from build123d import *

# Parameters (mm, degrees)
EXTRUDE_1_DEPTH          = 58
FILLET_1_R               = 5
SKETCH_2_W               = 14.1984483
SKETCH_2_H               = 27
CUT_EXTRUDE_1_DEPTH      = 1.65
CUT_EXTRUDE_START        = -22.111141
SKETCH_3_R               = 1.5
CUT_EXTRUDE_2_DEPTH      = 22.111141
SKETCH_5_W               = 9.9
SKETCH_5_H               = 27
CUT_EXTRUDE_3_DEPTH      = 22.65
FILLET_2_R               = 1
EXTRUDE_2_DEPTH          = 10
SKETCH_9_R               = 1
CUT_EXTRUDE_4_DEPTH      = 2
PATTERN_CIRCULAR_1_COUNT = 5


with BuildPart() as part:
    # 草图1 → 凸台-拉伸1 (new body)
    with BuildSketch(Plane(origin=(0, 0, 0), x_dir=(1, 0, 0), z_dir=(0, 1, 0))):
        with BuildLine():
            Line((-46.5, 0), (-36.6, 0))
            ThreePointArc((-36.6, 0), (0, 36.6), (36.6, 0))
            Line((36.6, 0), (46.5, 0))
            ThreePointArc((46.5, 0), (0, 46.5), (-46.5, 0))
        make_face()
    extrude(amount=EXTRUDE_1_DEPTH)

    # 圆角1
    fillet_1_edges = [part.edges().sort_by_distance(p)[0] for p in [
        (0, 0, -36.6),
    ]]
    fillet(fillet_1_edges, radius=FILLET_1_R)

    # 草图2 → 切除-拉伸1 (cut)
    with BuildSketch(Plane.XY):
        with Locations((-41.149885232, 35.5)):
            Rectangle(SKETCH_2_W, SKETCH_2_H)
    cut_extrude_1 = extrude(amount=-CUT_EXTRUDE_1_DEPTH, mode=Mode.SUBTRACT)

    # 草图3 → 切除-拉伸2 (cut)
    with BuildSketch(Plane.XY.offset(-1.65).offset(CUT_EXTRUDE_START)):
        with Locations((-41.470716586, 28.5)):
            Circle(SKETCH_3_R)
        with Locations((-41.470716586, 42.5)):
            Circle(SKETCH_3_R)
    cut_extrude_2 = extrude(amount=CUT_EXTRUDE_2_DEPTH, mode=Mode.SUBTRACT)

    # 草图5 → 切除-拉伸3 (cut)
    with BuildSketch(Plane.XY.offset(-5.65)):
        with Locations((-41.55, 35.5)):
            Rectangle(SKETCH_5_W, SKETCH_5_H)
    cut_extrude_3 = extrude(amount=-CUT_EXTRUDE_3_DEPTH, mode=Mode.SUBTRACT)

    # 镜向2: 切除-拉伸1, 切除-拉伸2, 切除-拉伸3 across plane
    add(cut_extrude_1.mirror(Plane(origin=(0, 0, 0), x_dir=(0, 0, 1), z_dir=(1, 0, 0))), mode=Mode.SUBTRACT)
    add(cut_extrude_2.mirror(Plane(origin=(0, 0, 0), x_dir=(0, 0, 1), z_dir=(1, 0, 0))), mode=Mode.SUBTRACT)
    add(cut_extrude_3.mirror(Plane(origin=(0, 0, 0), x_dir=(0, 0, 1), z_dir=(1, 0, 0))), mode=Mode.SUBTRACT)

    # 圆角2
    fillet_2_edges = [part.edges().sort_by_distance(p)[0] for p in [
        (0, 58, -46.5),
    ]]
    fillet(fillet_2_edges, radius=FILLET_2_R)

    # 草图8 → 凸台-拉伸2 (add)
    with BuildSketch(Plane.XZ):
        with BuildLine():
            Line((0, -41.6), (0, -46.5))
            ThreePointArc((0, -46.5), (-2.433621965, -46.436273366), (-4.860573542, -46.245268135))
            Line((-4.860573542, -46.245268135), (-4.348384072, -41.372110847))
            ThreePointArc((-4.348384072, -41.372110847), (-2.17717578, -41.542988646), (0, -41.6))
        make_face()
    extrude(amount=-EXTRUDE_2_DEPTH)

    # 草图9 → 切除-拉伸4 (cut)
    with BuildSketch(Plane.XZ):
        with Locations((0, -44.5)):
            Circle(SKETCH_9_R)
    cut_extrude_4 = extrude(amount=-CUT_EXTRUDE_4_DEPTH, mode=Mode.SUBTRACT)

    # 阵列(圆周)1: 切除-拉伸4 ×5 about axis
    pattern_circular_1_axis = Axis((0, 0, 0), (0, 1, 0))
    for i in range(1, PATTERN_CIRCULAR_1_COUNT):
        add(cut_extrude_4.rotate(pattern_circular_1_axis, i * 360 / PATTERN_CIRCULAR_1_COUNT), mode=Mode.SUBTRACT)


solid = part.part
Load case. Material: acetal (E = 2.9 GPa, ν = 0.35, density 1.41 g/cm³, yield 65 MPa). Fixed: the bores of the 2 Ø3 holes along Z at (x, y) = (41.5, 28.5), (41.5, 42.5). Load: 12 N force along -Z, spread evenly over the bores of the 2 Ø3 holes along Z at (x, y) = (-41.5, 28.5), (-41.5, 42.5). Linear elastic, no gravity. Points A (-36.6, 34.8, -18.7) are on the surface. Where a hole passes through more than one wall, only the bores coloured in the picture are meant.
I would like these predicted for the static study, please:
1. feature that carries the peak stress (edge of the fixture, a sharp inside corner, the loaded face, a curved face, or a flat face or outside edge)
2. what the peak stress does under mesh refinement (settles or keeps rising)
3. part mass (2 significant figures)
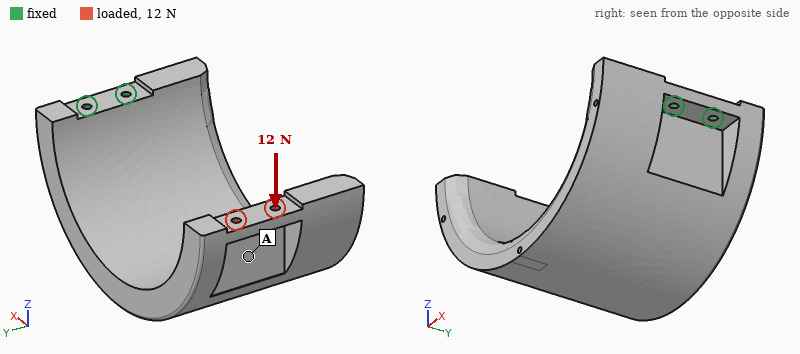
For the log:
edge of the fixture
keeps rising
93 g
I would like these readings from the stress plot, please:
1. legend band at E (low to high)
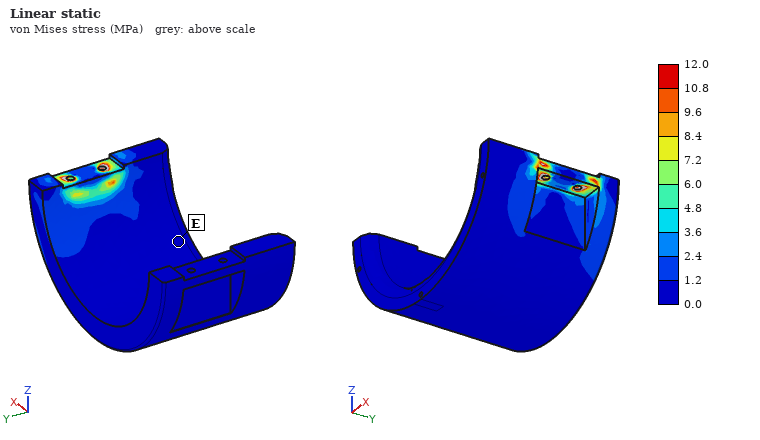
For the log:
0.0 to 1.2 MPa
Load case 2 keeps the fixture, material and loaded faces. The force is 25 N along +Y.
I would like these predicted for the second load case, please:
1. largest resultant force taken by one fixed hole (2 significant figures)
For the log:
100 N
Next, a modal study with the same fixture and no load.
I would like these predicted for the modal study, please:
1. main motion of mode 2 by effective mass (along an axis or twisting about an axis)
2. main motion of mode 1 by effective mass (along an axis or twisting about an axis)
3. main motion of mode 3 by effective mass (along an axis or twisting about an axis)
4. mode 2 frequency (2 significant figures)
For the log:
along Y
along Z
along Y
150 Hz
